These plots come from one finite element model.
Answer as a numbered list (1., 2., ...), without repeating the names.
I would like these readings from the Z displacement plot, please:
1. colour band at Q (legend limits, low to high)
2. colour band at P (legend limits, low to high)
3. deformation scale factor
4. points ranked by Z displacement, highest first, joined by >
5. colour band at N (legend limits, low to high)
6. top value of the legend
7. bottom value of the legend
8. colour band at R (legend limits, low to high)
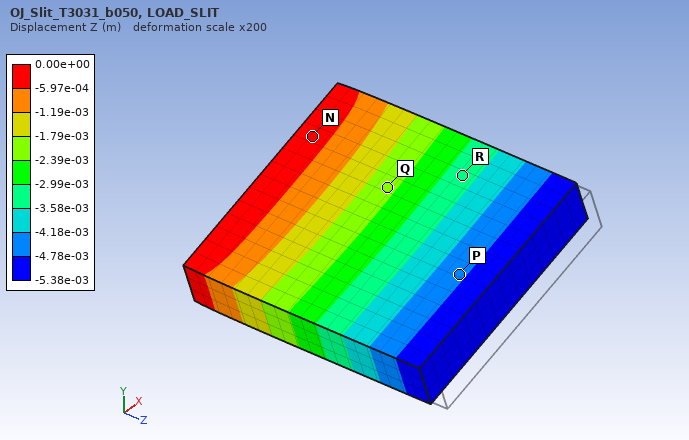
1. -2.39e-03 to -1.79e-03 m
2. -4.78e-03 to -4.18e-03 m
3. 200
4. N > Q > R > P
5. -5.97e-04 to 0.00e+00 m
6. 0.00e+00 m
7. -5.38e-03 m
8. -3.58e-03 to -2.99e-03 m
